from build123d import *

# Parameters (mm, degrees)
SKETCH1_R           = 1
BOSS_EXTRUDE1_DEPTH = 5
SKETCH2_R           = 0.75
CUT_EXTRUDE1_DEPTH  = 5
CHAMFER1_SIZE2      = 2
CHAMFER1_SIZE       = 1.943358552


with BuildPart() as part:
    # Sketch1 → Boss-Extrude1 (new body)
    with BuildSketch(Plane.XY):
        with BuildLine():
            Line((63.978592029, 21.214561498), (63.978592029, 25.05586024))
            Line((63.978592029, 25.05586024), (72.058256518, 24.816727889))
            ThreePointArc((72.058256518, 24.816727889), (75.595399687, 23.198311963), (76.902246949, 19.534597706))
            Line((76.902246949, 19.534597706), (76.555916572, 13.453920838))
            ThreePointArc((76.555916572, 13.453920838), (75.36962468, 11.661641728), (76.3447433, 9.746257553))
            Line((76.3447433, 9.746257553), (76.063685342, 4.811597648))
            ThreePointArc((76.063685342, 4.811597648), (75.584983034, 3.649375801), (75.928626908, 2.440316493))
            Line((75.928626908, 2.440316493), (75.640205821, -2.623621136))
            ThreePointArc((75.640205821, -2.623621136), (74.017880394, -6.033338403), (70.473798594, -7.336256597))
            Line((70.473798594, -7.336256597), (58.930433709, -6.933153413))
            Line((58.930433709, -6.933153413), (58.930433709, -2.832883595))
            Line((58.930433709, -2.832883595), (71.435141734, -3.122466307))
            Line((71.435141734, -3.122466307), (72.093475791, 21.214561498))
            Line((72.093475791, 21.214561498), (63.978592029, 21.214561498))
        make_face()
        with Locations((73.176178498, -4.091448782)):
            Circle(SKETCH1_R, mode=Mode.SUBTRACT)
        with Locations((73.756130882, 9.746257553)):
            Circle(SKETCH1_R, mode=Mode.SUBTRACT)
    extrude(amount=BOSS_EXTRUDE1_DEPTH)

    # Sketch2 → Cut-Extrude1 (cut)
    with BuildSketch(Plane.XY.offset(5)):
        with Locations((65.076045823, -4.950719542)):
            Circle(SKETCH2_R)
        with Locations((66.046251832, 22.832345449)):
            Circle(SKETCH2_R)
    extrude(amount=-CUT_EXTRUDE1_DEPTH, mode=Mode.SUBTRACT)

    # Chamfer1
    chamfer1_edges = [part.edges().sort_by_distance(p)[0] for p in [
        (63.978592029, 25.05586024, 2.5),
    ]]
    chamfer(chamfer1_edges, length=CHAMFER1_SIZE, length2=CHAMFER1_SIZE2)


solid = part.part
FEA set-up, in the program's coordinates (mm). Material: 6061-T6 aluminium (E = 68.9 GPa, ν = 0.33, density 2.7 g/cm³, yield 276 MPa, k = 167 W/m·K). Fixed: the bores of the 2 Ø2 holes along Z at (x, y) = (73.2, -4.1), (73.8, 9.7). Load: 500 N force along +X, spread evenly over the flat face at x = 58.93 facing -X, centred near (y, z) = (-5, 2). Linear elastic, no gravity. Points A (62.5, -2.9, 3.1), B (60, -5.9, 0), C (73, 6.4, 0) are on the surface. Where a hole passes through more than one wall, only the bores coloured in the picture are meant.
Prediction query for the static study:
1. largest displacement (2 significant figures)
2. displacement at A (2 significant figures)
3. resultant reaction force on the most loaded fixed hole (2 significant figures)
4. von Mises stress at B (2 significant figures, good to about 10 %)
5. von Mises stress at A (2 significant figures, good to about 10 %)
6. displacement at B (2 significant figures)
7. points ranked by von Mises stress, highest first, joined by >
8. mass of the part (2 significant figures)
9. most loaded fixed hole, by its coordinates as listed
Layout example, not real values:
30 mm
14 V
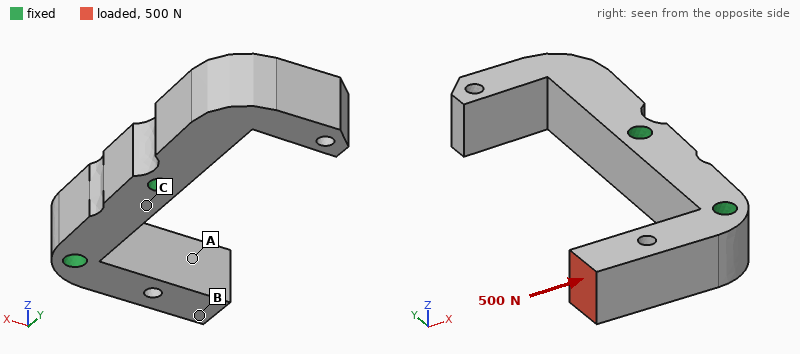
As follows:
6.1 µm
4.8 µm
500 N
24 MPa
32 MPa
5.3 µm
A > B > C
2.7 g
(73.2, -4.1)
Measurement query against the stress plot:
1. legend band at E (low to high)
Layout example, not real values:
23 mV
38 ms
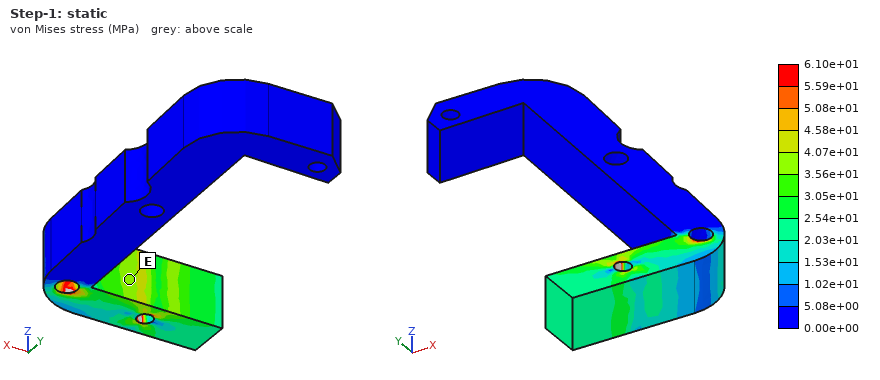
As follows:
3.56e+01 to 4.07e+01 MPa
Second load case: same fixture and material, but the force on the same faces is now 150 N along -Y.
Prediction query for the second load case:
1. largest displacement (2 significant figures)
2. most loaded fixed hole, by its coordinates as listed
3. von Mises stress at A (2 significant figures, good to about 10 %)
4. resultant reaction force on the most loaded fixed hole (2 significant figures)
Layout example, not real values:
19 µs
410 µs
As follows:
85 µm
(73.2, -4.1)
36 MPa
130 N
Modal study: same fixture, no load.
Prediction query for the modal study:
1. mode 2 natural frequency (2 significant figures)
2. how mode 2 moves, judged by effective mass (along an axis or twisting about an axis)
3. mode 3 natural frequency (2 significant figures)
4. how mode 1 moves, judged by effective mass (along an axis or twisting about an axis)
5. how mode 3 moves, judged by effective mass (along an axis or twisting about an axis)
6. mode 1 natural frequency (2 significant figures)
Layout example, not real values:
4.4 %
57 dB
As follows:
10 kHz
along Z
15 kHz
along X
along Y
8200 Hz
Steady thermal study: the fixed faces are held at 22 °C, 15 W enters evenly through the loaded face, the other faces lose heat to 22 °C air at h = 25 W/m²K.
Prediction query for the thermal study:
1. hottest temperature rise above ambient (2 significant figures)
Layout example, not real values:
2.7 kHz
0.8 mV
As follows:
63 K
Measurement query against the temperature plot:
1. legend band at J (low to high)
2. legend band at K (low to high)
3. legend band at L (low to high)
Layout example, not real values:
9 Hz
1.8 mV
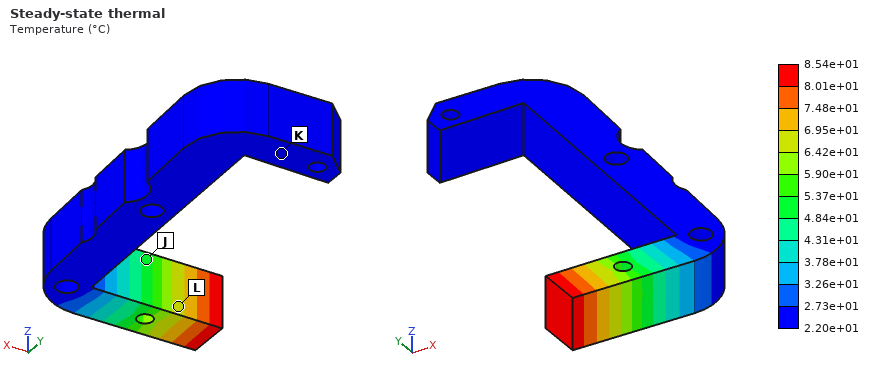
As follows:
4.84e+01 to 5.37e+01 °C
2.20e+01 to 2.73e+01 °C
6.42e+01 to 6.95e+01 °C
